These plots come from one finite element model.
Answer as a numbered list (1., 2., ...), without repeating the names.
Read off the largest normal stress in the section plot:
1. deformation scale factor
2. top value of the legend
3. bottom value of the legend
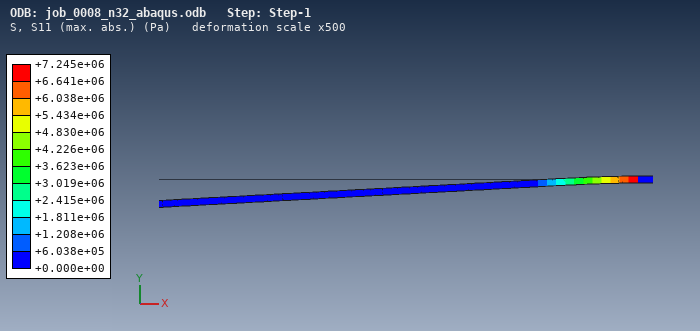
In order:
1. 500
2. +7.245e+06 Pa
3. +0.000e+00 Pa
